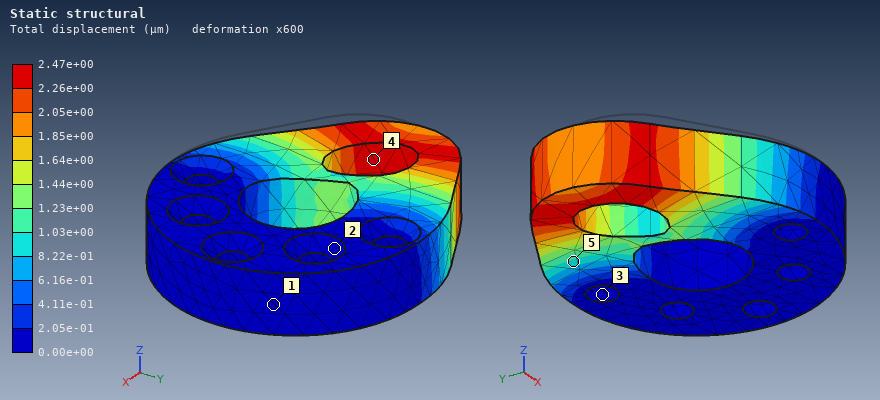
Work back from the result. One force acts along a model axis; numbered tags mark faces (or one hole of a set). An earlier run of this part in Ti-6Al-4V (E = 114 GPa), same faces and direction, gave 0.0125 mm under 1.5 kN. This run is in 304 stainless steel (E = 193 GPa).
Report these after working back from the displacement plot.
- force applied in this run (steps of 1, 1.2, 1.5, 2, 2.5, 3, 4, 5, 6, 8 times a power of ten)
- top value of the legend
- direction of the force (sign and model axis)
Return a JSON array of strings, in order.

["500 N", "2.47e+00 µm", "+Y"]
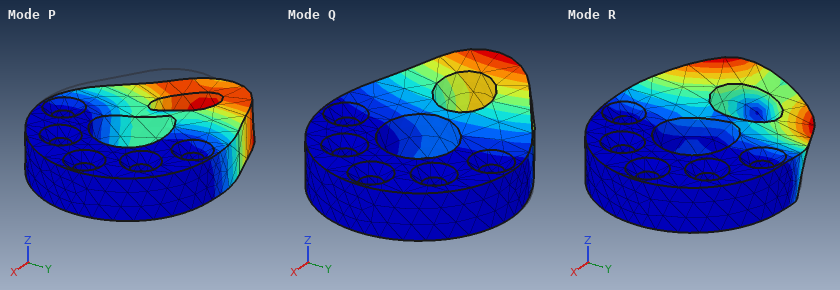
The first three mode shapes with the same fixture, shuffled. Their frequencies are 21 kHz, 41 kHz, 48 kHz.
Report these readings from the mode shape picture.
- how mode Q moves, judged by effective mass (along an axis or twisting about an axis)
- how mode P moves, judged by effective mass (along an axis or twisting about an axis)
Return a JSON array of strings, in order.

["along Z", "along Y"]
